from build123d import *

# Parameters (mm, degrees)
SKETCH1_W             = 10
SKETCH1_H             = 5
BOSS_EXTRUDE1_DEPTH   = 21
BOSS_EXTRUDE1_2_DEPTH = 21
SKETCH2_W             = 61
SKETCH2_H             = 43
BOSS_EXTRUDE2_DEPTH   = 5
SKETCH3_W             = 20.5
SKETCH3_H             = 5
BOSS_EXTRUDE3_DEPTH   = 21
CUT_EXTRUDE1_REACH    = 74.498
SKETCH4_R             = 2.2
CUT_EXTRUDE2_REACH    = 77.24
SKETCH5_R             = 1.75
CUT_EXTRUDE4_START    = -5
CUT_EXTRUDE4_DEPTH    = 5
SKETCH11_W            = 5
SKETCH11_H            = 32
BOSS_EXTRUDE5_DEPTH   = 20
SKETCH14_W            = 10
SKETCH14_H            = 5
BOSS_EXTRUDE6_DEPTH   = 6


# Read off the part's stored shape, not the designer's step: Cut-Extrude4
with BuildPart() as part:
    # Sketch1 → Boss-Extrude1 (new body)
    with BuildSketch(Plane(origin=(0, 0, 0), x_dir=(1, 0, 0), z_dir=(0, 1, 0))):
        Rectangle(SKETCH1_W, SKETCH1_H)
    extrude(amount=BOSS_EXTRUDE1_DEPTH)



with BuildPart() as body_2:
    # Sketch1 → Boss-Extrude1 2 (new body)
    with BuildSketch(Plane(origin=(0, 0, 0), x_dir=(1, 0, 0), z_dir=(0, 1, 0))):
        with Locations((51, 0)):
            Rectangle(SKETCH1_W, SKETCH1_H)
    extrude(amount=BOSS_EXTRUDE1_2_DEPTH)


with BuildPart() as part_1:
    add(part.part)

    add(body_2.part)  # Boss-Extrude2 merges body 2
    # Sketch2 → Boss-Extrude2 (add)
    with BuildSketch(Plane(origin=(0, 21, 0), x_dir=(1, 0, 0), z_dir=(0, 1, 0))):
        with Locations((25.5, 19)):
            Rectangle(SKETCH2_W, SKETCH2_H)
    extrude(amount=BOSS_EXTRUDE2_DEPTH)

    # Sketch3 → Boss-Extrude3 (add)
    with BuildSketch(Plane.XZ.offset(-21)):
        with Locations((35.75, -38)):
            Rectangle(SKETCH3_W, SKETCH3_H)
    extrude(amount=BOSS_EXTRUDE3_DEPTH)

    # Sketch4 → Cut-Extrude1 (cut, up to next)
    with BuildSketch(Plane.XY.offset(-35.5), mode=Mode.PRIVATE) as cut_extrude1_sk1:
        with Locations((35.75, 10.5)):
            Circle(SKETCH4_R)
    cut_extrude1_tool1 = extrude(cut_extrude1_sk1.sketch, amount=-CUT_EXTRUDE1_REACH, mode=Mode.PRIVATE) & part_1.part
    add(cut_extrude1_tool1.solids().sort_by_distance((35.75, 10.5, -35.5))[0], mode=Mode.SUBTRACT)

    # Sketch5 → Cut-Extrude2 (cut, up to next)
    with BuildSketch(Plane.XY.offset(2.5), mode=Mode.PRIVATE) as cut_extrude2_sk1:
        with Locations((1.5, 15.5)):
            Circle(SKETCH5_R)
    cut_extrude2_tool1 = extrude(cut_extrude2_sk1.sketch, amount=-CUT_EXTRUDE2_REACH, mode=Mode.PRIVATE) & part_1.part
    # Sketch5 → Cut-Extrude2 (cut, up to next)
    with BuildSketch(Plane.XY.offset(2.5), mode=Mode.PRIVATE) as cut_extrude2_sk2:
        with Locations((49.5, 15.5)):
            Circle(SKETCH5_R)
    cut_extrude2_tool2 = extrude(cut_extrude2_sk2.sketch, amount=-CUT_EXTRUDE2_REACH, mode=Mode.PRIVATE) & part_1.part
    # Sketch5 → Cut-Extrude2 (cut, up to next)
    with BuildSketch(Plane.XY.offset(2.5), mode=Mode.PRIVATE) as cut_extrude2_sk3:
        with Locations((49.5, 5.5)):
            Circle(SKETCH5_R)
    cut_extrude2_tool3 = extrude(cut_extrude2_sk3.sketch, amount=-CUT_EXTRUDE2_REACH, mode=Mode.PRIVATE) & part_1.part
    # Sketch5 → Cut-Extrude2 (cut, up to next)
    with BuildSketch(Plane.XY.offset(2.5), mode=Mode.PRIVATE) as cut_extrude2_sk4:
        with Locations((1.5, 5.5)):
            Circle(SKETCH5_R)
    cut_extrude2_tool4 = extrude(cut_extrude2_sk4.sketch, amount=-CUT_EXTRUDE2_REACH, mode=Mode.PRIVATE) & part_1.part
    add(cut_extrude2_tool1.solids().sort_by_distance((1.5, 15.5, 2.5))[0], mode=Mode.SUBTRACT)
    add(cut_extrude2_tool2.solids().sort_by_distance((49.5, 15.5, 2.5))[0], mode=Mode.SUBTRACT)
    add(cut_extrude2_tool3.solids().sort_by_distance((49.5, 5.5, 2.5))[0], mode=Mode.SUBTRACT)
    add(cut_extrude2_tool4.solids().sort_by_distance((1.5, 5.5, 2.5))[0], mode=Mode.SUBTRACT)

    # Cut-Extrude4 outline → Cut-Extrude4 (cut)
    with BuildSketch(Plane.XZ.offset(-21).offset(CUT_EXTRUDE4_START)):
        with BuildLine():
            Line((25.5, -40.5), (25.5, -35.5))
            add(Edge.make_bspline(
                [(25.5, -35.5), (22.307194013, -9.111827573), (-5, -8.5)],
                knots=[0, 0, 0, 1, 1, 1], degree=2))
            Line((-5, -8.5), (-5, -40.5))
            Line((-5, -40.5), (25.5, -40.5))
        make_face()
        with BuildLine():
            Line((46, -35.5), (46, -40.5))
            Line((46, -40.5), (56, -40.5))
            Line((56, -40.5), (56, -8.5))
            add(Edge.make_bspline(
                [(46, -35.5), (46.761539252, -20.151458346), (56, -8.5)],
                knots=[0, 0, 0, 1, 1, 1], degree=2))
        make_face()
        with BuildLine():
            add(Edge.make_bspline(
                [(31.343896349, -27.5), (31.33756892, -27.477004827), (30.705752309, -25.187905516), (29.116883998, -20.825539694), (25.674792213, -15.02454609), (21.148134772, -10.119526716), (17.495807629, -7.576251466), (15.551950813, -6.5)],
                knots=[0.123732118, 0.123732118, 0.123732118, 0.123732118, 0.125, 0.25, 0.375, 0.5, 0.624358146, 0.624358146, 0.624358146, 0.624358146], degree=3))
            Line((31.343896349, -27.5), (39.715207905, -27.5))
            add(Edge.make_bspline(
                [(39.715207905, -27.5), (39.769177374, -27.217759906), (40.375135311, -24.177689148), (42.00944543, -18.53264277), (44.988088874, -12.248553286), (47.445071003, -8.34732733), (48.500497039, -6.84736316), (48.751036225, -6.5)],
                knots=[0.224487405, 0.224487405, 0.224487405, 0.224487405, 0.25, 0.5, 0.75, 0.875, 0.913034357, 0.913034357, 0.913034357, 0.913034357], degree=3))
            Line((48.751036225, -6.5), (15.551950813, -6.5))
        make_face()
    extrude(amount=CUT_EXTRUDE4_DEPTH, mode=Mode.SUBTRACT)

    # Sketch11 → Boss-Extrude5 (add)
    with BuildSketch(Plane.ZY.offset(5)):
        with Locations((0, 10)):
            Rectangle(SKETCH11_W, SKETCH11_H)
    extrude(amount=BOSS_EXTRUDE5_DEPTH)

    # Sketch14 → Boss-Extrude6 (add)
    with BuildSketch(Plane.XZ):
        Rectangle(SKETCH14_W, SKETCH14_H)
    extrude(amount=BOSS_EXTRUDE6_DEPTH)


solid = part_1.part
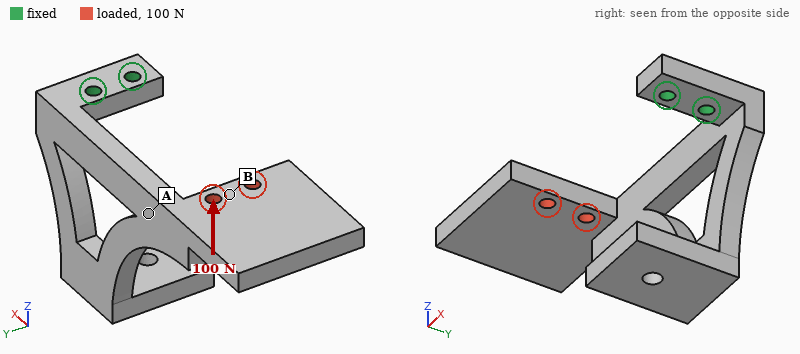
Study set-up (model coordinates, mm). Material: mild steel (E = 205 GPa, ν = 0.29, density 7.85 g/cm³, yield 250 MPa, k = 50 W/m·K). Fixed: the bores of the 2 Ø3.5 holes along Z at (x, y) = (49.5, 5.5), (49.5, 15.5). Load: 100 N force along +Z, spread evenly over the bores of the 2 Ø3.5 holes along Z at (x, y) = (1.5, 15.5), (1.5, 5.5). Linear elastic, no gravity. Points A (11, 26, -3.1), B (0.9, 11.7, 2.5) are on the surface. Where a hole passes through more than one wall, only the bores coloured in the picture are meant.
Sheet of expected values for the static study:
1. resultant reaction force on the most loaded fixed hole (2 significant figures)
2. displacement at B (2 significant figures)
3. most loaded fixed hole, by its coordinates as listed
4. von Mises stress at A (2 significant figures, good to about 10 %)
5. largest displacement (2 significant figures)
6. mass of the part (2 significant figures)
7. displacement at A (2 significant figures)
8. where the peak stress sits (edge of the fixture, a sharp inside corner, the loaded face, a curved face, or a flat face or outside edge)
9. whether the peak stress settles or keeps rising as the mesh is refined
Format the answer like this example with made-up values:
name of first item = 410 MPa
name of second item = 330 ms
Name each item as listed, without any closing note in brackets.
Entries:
resultant reaction force on the most loaded fixed hole = 69 N
displacement at B = 0.12 mm
most loaded fixed hole, by its coordinates as listed = (49.5, 15.5)
von Mises stress at A = 27 MPa
largest displacement = 0.21 mm
mass of the part = 110 g
displacement at A = 0.064 mm
where the peak stress sits = edge of the fixture
whether the peak stress settles or keeps rising as the mesh is refined = keeps rising
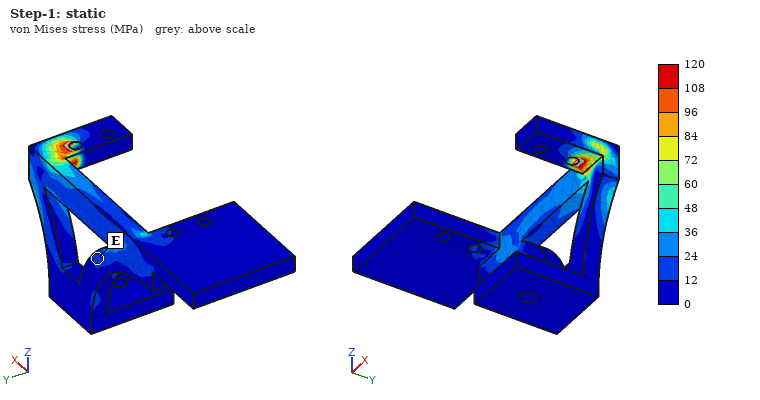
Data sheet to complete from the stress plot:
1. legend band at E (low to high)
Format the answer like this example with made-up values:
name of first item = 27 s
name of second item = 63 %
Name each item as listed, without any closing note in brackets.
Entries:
legend band at E = 12 to 24 MPa
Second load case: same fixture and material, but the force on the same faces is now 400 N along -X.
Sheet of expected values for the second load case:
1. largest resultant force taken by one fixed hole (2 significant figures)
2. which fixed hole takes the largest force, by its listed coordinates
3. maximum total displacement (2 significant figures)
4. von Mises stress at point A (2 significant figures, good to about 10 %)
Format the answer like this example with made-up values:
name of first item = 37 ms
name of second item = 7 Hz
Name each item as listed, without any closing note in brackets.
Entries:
largest resultant force taken by one fixed hole = 310 N
which fixed hole takes the largest force, by its listed coordinates = (49.5, 15.5)
maximum total displacement = 0.56 mm
von Mises stress at point A = 81 MPa
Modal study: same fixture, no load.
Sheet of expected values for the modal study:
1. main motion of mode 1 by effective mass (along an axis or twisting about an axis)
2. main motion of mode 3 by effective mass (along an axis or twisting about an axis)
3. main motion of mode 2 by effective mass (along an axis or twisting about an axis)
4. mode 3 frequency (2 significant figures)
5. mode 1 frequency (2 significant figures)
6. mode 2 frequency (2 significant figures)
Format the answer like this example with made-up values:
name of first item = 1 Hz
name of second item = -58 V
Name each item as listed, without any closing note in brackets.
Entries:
main motion of mode 1 by effective mass = along Y
main motion of mode 3 by effective mass = along Y
main motion of mode 2 by effective mass = along Z
mode 3 frequency = 790 Hz
mode 1 frequency = 410 Hz
mode 2 frequency = 530 Hz
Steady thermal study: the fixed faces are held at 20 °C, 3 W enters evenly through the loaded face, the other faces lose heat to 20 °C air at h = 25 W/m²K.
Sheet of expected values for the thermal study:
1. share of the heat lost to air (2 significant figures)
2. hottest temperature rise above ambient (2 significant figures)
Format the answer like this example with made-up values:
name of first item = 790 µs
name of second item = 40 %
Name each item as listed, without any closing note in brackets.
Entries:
share of the heat lost to air = 74 %
hottest temperature rise above ambient = 27 K
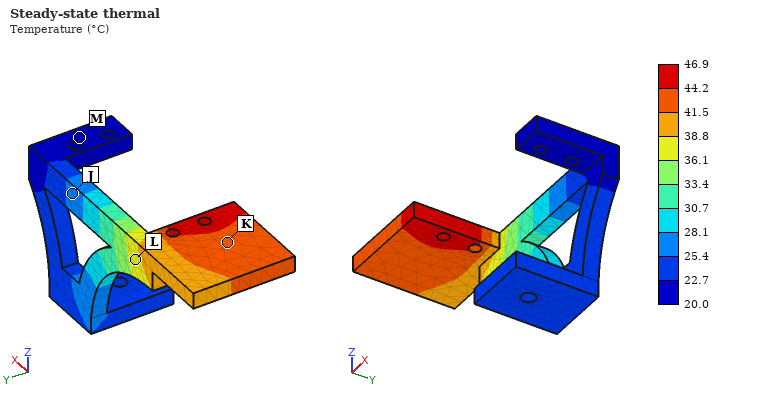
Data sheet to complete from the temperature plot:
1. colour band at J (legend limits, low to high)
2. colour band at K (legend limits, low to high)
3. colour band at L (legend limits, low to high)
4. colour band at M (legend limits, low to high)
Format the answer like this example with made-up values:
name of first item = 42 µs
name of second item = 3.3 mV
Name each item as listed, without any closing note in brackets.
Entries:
colour band at J = 25.4 to 28.1 °C
colour band at K = 41.5 to 44.2 °C
colour band at L = 36.1 to 38.8 °C
colour band at M = 20.0 to 22.7 °C
